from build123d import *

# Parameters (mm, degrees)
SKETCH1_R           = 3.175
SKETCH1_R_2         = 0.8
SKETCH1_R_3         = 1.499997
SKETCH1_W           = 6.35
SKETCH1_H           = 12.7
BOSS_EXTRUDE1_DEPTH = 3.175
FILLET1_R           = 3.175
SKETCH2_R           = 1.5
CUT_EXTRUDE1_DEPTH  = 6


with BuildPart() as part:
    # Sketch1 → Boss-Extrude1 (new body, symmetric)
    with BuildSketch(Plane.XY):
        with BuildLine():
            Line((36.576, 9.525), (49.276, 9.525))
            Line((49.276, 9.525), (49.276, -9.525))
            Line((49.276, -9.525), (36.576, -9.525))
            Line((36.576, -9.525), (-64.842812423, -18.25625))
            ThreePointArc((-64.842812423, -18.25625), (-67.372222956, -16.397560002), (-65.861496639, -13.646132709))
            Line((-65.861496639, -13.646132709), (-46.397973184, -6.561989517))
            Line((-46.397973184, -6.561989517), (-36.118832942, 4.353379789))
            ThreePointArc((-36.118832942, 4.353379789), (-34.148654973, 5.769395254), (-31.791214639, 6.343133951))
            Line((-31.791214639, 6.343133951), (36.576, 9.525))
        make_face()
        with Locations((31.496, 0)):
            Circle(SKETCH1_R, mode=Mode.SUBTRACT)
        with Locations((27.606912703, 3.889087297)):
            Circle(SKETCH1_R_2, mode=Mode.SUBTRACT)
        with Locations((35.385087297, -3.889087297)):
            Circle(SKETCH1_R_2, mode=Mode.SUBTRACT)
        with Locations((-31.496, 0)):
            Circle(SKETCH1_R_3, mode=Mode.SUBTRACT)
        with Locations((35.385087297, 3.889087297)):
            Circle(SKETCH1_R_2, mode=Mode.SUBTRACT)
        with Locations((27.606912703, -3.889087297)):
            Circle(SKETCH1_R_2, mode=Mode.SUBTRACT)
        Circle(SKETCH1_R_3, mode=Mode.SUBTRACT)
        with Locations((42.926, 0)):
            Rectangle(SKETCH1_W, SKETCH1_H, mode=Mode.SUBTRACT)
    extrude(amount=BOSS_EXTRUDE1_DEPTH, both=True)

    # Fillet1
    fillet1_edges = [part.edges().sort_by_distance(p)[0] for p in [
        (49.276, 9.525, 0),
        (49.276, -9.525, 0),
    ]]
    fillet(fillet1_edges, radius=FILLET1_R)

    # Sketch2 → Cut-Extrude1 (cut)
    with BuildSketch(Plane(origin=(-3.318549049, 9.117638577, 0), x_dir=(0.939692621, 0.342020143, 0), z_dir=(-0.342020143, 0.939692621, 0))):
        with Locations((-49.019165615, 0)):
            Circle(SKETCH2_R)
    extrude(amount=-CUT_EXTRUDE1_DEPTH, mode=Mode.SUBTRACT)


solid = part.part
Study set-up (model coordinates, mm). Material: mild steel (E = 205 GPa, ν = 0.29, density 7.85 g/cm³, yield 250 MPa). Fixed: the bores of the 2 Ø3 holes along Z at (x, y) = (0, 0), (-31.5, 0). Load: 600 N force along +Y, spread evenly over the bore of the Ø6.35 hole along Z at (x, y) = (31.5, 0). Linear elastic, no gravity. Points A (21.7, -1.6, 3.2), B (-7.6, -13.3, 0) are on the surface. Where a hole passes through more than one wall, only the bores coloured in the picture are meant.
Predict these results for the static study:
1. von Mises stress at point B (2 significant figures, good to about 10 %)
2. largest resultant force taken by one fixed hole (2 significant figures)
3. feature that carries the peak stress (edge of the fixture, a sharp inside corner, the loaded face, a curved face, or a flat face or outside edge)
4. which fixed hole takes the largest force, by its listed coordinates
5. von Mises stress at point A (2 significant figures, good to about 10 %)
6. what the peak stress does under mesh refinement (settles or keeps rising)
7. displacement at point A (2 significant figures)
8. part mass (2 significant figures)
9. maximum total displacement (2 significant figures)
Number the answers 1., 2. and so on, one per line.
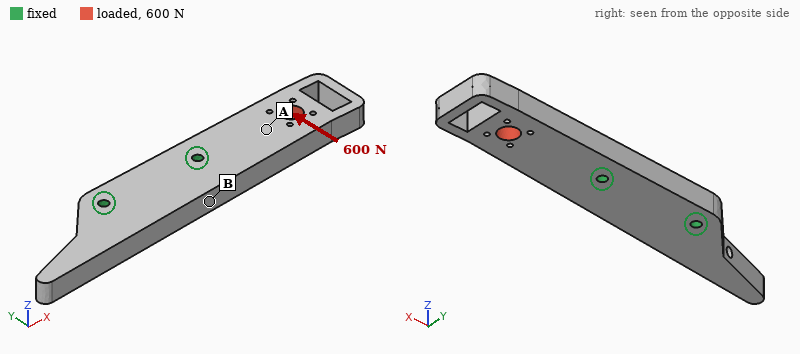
1. 27 MPa
2. 1.2 kN
3. edge of the fixture
4. (0, 0)
5. 14 MPa
6. keeps rising
7. 10 µm
8. 94 g
9. 27 µm
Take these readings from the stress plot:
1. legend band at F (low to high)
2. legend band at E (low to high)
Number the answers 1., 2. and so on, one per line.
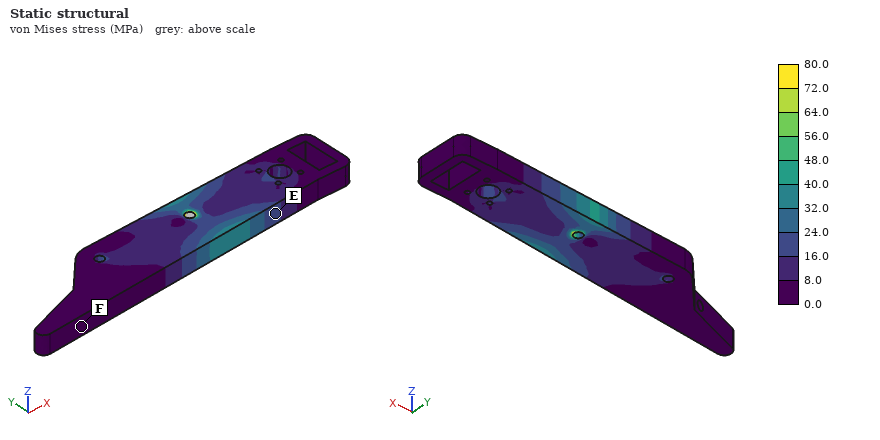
1. 0.0 to 8.0 MPa
2. 16.0 to 24.0 MPa
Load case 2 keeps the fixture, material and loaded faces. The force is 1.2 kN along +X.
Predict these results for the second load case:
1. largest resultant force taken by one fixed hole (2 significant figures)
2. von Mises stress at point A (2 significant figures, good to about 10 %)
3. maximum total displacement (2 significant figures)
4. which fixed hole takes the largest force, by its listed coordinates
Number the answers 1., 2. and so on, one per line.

1. 1.1 kN
2. 10 MPa
3. 3.4 µm
4. (0, 0)
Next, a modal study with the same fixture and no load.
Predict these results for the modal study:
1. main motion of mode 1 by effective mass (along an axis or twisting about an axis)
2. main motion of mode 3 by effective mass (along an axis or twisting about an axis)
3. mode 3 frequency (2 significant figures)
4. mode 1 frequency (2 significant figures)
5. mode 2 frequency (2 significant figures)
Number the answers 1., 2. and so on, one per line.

1. along Z
2. along Y
3. 5500 Hz
4. 2400 Hz
5. 4800 Hz
